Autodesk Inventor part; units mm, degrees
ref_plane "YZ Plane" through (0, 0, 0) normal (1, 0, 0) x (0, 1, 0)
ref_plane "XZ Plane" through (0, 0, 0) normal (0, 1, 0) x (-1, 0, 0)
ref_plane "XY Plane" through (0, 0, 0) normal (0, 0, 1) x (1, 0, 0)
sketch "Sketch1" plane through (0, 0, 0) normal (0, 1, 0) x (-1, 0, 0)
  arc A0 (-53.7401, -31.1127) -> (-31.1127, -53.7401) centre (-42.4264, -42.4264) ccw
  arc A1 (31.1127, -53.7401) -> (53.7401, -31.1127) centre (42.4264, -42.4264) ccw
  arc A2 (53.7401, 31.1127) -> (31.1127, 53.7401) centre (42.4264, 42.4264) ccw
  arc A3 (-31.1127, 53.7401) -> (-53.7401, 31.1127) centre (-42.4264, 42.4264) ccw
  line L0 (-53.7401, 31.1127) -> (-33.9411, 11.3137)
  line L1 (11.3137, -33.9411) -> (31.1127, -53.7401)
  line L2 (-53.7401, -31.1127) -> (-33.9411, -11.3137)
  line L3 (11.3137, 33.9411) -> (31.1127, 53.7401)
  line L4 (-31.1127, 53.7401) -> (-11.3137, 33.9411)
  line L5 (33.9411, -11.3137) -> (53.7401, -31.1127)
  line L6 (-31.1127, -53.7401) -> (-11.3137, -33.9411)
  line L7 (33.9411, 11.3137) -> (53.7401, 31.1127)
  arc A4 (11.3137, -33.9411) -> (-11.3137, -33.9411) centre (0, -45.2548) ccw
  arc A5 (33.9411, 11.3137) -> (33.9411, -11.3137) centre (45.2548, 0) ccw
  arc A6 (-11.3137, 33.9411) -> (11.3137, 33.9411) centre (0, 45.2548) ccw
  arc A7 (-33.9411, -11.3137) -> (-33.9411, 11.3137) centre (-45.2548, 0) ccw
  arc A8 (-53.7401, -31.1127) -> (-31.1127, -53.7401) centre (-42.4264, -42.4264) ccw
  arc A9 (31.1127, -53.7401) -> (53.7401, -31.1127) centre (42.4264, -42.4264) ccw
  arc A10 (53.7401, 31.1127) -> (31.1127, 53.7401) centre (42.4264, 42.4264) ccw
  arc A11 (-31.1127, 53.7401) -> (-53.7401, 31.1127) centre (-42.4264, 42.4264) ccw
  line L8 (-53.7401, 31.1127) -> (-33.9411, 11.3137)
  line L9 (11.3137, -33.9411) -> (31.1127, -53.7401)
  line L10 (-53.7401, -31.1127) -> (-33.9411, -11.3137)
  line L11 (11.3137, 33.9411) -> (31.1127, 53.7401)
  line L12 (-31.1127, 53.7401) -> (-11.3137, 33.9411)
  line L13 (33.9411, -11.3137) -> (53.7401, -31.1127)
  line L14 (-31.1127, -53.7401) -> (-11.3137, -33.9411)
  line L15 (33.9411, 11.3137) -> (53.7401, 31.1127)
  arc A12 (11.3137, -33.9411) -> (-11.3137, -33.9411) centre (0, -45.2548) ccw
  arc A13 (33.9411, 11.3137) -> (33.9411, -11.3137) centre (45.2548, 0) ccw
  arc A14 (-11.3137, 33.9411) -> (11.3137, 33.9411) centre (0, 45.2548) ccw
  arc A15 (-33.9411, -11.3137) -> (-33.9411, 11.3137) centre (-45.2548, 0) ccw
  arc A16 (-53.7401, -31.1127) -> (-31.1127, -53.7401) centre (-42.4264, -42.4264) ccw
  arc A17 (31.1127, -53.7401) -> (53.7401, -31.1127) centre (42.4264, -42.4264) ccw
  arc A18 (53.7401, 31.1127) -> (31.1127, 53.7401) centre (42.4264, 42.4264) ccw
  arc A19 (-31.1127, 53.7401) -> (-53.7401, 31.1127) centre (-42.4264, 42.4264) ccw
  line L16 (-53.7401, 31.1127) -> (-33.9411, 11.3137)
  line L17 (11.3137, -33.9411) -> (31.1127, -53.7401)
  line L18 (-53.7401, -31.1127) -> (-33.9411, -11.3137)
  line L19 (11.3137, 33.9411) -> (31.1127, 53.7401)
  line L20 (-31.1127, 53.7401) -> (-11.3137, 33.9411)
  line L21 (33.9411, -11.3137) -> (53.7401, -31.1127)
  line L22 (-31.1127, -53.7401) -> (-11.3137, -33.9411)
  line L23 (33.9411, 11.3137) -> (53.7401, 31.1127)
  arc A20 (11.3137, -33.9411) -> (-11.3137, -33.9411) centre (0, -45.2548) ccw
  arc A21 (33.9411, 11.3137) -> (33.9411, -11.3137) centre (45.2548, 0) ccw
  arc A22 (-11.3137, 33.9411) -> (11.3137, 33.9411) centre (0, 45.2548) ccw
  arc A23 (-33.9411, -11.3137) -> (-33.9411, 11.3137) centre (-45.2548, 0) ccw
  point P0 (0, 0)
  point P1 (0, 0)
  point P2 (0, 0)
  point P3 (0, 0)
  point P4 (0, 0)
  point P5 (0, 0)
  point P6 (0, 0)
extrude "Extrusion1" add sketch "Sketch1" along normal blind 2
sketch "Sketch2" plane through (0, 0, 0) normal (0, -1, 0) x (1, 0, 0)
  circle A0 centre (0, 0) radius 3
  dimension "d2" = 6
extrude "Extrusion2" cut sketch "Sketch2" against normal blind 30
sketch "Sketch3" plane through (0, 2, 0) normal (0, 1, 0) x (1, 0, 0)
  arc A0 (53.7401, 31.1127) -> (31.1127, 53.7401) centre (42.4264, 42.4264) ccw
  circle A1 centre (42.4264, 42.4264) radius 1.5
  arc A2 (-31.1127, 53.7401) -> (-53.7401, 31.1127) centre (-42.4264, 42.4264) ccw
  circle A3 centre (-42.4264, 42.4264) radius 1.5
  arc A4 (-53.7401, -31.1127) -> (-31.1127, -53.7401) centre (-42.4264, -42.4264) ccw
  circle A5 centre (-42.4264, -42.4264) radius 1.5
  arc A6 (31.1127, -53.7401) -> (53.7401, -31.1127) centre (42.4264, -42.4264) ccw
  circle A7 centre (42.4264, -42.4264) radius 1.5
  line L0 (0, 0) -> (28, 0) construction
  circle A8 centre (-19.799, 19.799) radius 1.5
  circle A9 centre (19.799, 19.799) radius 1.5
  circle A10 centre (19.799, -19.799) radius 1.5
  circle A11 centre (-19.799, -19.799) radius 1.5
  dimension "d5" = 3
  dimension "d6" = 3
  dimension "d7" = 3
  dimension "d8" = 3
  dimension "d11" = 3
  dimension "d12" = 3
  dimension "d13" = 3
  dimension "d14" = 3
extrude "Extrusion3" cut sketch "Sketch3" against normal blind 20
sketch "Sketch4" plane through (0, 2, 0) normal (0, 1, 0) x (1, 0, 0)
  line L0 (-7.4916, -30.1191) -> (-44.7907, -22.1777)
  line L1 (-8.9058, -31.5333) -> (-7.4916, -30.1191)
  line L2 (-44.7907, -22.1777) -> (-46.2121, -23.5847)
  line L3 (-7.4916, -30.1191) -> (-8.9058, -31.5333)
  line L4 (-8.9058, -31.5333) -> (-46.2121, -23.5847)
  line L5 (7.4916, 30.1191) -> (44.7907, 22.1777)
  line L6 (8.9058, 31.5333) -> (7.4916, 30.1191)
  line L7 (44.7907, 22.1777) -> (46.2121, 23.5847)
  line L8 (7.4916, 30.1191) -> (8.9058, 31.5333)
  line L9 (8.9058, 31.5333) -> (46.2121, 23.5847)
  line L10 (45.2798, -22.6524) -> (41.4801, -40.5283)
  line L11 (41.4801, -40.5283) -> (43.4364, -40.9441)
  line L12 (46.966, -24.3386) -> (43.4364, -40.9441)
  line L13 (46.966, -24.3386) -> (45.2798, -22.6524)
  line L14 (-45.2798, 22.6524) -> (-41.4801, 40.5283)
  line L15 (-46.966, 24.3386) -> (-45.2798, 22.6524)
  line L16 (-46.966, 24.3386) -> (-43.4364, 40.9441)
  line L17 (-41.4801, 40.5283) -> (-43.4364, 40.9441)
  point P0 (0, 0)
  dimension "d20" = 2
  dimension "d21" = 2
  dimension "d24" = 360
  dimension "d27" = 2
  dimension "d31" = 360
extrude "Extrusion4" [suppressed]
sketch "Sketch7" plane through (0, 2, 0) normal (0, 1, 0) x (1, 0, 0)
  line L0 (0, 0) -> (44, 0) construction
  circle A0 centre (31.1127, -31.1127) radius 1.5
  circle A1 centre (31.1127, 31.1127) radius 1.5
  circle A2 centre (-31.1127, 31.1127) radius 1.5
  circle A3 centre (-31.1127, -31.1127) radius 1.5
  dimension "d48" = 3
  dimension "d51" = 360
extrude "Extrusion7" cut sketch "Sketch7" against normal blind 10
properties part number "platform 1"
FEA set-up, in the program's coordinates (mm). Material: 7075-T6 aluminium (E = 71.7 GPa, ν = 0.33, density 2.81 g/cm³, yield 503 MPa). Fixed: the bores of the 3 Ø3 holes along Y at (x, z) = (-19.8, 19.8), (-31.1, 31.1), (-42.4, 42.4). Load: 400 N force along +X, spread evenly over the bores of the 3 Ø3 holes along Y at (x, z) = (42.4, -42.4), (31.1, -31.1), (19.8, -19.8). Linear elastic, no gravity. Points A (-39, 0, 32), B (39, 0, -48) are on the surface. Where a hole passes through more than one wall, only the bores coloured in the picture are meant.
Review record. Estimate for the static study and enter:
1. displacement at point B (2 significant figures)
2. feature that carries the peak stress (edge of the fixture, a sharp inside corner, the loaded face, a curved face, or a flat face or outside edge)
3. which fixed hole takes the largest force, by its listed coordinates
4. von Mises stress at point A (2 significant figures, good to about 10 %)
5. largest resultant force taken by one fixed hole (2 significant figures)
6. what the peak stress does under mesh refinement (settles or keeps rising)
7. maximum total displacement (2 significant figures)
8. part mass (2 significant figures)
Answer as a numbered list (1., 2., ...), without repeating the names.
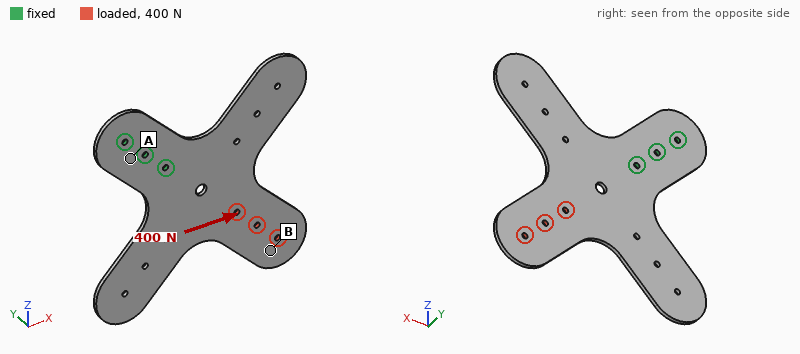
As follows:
1. 0.16 mm
2. edge of the fixture
3. (-19.8, 19.8)
4. 17 MPa
5. 1.0 kN
6. keeps rising
7. 0.19 mm
8. 47 g
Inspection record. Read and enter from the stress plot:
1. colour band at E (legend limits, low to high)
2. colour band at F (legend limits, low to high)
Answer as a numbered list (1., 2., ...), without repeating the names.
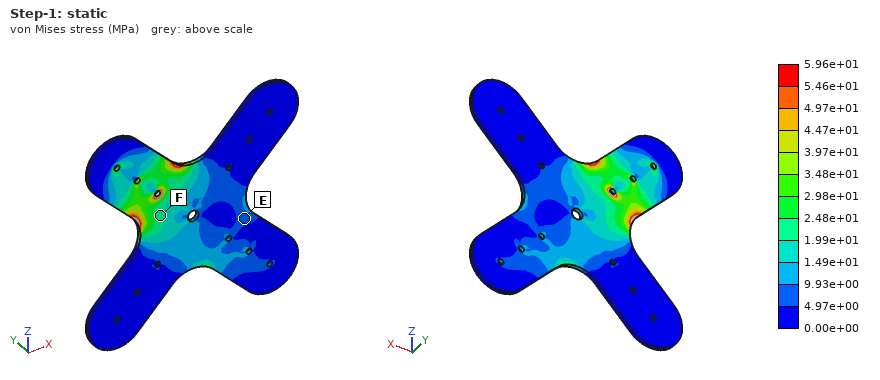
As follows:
1. 4.97e+00 to 9.93e+00 MPa
2. 1.99e+01 to 2.48e+01 MPa
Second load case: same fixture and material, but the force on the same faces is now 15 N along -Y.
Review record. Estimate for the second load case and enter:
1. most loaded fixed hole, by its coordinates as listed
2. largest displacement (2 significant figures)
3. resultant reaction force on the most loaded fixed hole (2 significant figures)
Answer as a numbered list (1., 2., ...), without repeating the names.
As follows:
1. (-19.8, 19.8)
2. 1.5 mm
3. 47 N
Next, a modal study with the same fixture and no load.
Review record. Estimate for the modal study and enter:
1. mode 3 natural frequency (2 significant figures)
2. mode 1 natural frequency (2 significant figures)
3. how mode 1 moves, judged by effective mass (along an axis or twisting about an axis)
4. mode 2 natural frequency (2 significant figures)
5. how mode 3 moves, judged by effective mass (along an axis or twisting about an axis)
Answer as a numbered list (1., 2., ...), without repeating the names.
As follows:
1. 370 Hz
2. 180 Hz
3. along Y
4. 230 Hz
5. along Y
